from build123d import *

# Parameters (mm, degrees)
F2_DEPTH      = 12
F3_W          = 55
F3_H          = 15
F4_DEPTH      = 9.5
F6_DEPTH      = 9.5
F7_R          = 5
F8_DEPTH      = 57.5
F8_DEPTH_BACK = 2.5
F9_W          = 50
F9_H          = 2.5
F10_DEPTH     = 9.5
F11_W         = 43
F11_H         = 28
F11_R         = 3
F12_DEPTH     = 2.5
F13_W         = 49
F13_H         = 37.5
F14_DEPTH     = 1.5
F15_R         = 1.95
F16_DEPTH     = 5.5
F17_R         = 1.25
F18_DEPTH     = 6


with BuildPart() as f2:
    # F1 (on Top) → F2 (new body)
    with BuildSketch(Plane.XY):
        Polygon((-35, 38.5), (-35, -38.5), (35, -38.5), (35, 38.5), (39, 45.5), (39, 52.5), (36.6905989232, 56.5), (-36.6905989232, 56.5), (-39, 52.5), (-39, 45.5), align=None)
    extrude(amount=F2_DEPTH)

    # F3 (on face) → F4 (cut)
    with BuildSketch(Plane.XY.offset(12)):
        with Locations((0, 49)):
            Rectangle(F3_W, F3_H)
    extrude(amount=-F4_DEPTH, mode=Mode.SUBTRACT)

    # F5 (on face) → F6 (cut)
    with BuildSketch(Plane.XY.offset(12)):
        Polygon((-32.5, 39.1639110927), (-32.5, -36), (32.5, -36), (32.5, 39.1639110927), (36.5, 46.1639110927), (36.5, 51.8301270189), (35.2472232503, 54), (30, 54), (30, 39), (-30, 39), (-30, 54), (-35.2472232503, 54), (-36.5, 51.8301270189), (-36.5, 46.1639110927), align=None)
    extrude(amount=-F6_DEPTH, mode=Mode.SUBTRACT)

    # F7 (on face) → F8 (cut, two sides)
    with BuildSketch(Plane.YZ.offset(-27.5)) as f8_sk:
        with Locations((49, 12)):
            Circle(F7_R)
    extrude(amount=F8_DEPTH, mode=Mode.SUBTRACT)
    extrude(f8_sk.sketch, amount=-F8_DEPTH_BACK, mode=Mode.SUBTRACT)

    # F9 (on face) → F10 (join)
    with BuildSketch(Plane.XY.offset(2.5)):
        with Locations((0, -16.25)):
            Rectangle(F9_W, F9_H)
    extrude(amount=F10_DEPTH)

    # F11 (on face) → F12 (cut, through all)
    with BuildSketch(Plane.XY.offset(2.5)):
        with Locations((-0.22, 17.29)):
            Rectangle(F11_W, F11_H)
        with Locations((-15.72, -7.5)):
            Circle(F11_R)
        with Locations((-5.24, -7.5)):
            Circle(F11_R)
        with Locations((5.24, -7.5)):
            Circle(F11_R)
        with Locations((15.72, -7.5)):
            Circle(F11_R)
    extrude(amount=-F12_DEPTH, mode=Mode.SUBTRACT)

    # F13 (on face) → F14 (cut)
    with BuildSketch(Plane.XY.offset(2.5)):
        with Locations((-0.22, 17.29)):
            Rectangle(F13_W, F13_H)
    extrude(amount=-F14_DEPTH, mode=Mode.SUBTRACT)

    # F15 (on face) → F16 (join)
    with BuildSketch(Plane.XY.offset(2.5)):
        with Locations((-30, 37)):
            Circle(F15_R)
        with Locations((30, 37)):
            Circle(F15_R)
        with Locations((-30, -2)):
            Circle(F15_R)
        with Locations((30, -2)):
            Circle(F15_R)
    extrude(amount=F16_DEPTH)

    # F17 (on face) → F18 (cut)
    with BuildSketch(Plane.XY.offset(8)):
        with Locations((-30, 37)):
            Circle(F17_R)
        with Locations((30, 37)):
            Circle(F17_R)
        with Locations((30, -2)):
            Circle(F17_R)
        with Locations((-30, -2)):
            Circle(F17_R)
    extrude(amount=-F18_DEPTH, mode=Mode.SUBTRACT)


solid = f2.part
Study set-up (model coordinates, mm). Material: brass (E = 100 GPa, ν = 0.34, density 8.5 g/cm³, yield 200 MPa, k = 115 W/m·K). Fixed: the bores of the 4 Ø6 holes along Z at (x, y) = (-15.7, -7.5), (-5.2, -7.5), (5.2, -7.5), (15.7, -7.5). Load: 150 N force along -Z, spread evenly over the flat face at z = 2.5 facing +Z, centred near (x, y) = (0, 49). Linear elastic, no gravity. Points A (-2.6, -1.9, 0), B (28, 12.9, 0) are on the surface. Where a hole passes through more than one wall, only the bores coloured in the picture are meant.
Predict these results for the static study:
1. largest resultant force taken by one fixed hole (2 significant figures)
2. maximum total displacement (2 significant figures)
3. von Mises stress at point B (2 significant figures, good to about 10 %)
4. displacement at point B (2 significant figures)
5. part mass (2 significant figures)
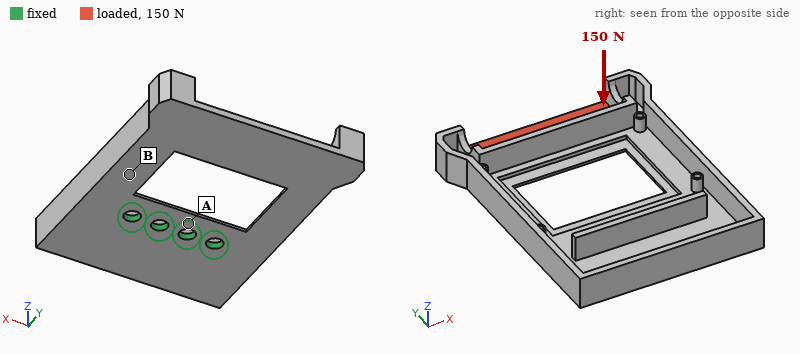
190 N
0.61 mm
31 MPa
0.18 mm
190 g
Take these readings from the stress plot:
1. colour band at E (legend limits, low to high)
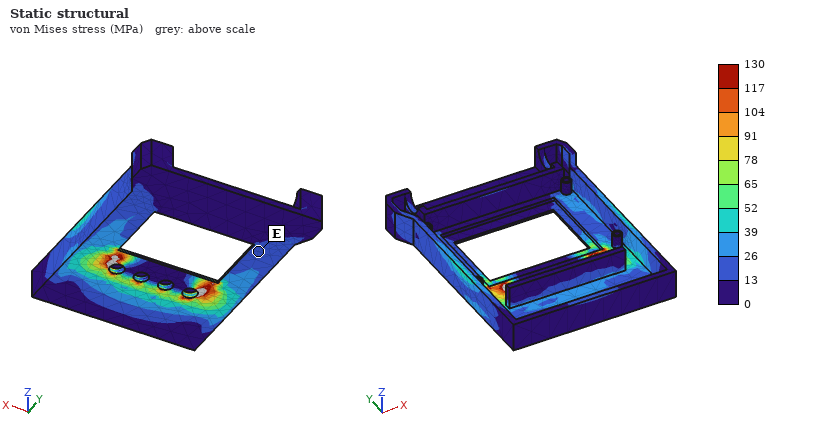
13 to 26 MPa
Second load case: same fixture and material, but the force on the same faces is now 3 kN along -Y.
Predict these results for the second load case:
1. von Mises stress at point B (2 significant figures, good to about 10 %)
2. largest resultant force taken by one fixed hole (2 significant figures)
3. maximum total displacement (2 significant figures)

44 MPa
1.6 kN
0.27 mm
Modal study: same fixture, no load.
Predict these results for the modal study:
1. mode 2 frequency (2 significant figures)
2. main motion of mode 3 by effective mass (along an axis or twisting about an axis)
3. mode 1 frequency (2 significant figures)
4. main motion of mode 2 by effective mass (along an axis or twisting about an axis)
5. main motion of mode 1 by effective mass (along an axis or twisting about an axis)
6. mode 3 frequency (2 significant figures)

510 Hz
along X
330 Hz
twisting about Y
along Z
1500 Hz
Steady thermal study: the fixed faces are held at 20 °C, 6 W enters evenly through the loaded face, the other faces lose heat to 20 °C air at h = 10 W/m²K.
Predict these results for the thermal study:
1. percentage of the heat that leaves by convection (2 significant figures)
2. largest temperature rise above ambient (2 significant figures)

32 %
26 K
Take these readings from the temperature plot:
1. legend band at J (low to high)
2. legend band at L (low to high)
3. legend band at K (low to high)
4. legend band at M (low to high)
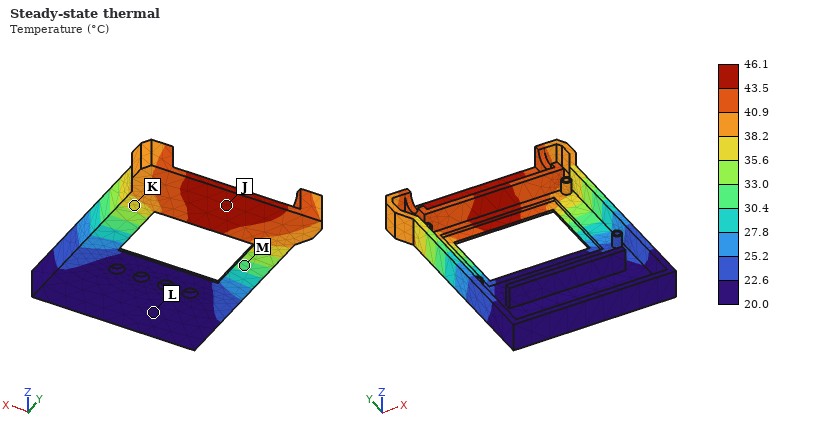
43.5 to 46.1 °C
20.0 to 22.6 °C
35.6 to 38.2 °C
30.4 to 33.0 °C
